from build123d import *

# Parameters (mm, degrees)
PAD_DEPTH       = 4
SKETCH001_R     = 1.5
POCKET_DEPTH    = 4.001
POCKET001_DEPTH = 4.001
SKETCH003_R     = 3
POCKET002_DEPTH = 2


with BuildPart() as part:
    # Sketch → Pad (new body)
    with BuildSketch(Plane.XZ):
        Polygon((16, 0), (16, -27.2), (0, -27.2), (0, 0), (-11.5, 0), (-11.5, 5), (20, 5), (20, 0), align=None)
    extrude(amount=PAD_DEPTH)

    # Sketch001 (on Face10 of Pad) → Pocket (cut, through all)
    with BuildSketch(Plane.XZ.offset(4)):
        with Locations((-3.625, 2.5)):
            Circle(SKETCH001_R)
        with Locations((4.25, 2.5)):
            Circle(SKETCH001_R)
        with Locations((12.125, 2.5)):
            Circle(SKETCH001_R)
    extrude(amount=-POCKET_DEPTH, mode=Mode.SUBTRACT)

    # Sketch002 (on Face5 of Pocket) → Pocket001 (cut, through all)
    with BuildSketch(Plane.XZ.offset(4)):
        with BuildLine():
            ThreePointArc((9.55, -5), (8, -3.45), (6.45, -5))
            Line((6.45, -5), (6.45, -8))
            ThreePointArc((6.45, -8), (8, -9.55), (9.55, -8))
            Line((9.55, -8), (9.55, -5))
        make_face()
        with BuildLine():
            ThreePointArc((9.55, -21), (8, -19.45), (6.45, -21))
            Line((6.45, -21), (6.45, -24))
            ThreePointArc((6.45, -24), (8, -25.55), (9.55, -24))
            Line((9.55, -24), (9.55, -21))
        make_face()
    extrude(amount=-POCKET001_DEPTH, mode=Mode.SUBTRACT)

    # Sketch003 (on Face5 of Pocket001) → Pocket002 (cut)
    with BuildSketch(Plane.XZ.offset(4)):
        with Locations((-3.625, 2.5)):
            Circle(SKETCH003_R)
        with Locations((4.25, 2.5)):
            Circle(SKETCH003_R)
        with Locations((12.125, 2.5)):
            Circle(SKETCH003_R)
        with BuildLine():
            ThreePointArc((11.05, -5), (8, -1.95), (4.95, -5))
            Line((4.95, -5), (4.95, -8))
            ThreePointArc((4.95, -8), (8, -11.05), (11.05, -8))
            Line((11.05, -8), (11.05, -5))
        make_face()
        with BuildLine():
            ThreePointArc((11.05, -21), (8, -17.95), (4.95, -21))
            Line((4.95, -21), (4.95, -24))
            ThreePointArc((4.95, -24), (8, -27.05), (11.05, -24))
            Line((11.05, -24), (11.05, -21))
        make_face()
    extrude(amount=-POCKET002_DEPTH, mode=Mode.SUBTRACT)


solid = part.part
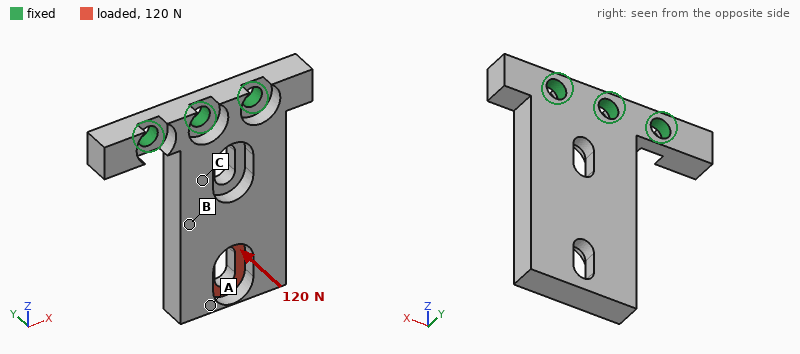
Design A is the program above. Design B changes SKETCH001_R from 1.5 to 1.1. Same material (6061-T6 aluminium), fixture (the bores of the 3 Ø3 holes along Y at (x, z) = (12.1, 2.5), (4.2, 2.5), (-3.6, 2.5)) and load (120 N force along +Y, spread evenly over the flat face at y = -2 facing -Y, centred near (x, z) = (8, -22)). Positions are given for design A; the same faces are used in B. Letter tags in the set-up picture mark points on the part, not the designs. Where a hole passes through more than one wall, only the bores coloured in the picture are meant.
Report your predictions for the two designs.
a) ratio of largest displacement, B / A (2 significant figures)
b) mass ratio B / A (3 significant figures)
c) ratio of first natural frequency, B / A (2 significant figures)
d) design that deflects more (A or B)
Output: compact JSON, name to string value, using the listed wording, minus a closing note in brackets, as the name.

{"ratio of largest displacement, B / A": "1.1", "mass ratio B / A": "1.01", "ratio of first natural frequency, B / A": "0.92", "design that deflects more": "B"}
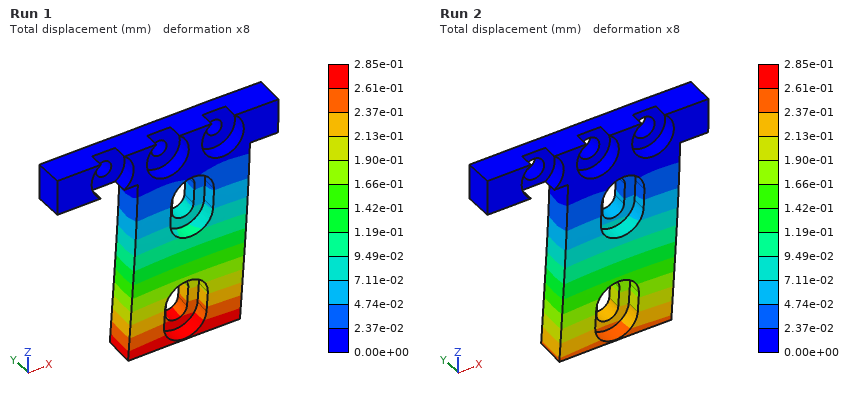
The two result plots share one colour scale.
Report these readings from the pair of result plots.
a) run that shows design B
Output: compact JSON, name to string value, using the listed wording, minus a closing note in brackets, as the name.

{"run that shows design B": "Run 1"}
